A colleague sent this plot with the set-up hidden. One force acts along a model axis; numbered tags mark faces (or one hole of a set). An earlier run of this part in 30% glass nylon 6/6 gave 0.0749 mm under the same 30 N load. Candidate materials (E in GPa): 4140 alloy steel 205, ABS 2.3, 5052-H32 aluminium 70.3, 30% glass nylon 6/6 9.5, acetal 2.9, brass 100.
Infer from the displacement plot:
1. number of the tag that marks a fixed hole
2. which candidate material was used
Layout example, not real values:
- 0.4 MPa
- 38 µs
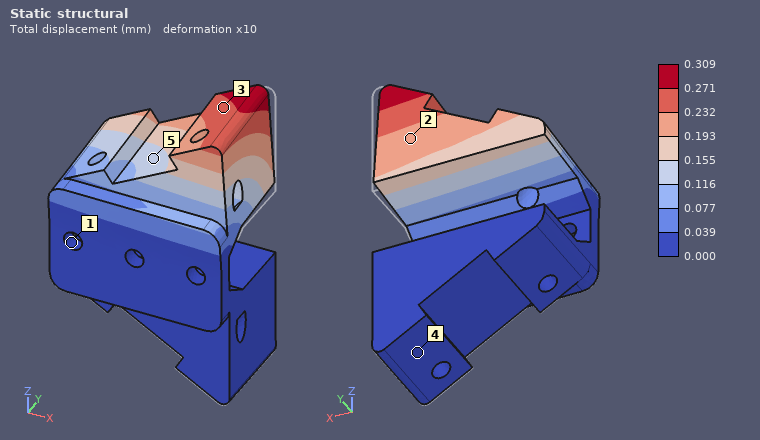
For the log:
- 1
- ABS
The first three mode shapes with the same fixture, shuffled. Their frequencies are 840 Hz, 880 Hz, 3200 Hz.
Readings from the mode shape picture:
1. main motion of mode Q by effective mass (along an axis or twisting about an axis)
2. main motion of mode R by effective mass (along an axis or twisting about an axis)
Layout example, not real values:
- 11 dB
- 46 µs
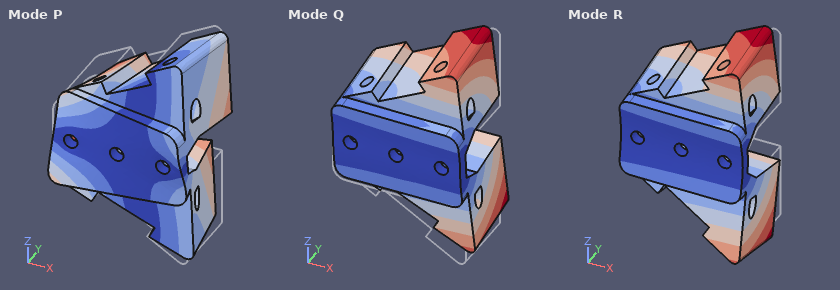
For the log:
- along Z
- along Y
